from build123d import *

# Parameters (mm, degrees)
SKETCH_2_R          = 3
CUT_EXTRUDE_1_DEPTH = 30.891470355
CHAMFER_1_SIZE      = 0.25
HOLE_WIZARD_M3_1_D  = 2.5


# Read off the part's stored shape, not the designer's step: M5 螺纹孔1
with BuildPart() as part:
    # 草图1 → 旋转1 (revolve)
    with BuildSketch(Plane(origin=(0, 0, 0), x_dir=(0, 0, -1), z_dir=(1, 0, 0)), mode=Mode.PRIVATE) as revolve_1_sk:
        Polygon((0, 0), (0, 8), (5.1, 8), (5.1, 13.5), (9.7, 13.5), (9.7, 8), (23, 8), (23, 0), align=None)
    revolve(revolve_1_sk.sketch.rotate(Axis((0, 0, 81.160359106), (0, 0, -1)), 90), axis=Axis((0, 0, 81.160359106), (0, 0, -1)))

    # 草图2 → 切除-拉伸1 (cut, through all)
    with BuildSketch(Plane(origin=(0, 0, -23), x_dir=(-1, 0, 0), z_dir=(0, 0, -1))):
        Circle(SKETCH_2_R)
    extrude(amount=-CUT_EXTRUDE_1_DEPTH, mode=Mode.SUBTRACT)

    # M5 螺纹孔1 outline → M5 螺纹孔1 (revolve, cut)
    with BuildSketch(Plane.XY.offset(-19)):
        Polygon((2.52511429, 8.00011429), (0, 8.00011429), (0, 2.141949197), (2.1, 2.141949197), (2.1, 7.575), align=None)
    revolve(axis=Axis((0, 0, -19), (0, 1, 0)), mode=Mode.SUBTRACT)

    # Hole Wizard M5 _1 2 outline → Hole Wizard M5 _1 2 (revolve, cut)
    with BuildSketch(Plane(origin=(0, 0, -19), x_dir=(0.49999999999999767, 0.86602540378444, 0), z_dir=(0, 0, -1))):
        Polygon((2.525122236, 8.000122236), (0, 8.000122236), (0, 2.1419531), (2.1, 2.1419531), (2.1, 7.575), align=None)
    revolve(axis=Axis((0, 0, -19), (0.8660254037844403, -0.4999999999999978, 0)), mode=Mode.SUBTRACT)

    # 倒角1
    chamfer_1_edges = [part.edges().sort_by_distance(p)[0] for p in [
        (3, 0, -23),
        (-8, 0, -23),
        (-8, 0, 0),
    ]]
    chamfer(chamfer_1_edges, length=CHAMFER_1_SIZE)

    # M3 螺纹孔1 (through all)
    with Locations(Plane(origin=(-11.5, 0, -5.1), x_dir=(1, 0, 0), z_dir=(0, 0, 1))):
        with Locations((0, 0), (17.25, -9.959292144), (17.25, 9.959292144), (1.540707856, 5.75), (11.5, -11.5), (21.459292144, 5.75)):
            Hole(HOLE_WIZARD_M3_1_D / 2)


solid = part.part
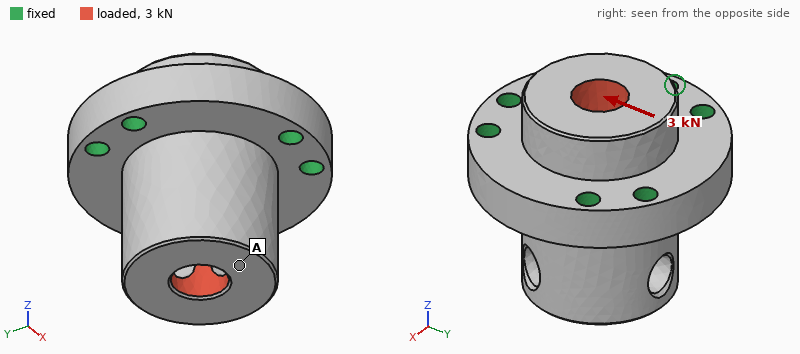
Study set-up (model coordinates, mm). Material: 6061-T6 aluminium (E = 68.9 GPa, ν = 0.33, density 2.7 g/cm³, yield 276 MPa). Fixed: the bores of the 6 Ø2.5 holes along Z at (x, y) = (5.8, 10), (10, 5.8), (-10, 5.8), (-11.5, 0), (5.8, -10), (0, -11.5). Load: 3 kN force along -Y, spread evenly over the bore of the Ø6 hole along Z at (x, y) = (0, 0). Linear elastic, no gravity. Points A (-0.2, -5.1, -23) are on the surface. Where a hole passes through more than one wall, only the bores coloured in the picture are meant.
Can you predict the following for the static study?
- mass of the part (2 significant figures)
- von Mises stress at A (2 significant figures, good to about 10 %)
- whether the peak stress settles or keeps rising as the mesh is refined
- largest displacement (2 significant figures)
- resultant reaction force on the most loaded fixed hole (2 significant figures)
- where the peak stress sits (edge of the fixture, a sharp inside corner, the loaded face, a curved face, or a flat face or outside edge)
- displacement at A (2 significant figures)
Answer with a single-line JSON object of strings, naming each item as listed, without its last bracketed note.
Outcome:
{"mass of the part": "15 g", "von Mises stress at A": "9.2 MPa", "whether the peak stress settles or keeps rising as the mesh is refined": "keeps rising", "largest displacement": "12 µm", "resultant reaction force on the most loaded fixed hole": "770 N", "where the peak stress sits": "edge of the fixture", "displacement at A": "12 µm"}
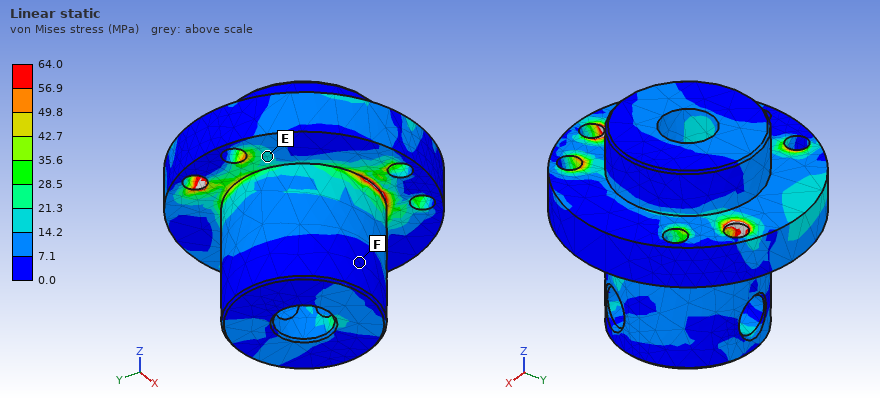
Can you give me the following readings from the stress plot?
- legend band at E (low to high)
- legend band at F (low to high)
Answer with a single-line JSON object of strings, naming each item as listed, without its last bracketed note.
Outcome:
{"legend band at E": "14.2 to 21.3 MPa", "legend band at F": "0.0 to 7.1 MPa"}
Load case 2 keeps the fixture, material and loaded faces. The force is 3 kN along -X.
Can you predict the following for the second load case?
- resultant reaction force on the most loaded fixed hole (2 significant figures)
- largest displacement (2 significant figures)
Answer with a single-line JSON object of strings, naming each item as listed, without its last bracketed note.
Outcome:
{"resultant reaction force on the most loaded fixed hole": "770 N", "largest displacement": "13 µm"}
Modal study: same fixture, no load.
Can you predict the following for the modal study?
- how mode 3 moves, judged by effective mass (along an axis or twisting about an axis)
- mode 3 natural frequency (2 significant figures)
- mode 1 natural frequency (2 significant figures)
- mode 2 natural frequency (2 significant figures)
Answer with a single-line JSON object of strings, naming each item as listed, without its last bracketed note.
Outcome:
{"how mode 3 moves, judged by effective mass": "along Z", "mode 3 natural frequency": "40 kHz", "mode 1 natural frequency": "26 kHz", "mode 2 natural frequency": "27 kHz"}
